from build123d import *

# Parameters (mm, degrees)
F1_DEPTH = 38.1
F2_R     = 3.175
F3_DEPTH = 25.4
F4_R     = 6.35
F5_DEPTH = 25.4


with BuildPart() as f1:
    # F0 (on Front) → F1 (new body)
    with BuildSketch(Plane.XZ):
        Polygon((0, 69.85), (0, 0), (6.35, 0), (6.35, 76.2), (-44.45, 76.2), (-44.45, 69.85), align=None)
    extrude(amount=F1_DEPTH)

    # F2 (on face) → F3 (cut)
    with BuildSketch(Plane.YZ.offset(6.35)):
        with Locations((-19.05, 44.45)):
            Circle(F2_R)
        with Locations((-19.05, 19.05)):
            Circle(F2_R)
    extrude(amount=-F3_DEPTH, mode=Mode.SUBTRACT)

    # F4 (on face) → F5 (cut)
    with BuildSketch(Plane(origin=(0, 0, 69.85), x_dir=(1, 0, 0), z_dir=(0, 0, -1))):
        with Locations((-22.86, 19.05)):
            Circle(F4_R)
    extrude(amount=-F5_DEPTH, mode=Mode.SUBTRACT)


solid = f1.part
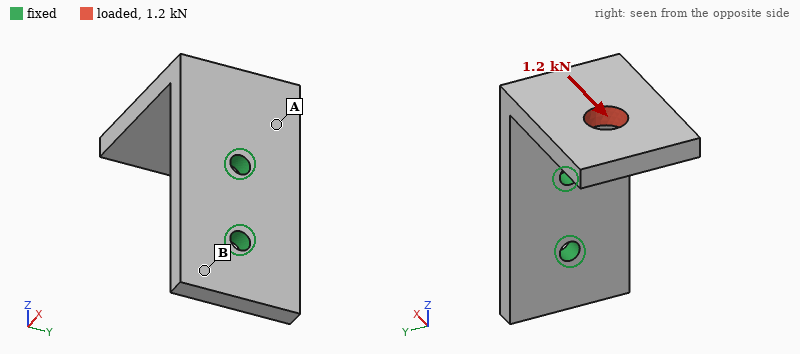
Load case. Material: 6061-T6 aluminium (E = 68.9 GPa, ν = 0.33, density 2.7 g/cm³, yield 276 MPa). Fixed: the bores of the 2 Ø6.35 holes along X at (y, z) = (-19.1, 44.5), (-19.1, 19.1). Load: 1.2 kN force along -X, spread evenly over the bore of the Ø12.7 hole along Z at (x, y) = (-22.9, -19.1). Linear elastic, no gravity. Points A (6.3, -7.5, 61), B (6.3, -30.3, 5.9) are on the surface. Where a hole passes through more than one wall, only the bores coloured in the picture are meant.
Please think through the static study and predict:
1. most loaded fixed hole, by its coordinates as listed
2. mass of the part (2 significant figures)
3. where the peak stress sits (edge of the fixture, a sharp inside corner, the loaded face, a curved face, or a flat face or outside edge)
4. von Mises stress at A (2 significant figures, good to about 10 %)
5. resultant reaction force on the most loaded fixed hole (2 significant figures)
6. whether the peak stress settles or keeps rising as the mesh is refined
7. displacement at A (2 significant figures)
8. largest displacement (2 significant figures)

(-19.1, 44.5)
76 g
edge of the fixture
52 MPa
1.6 kN
keeps rising
0.080 mm
0.46 mm
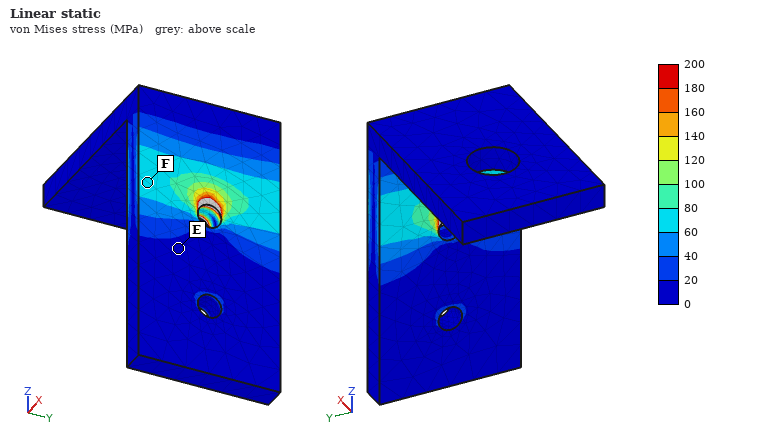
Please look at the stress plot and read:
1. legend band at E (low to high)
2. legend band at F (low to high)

0 to 20 MPa
60 to 80 MPa
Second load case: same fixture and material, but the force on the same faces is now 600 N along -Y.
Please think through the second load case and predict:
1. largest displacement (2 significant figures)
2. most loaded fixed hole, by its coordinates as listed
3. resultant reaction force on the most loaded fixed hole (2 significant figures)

0.26 mm
(-19.1, 44.5)
1.1 kN
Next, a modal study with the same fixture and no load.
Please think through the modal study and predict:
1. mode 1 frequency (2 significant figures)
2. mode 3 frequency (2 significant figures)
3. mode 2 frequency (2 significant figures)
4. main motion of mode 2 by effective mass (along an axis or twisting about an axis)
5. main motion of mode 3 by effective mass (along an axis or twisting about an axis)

1200 Hz
3500 Hz
1700 Hz
along Y
along X
